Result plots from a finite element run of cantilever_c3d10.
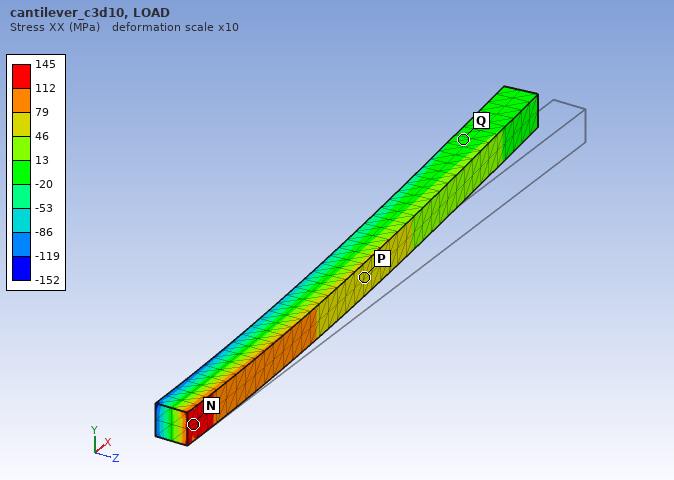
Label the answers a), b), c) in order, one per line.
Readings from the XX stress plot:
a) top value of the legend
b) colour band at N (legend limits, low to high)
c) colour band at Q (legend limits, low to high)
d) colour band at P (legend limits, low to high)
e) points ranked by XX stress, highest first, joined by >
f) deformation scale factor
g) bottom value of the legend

a) 145 MPa
b) 112 to 145 MPa
c) -20 to 13 MPa
d) 46 to 79 MPa
e) N > P > Q
f) 10
g) -152 MPa
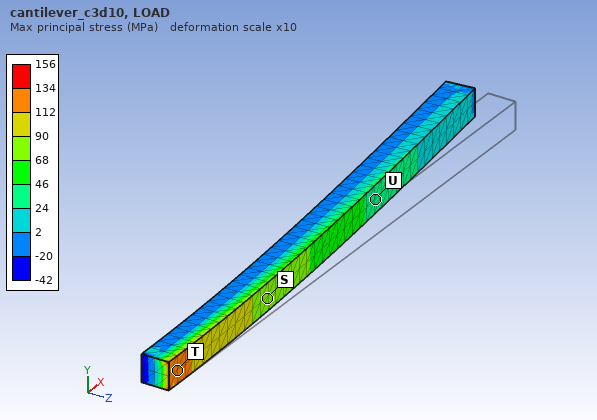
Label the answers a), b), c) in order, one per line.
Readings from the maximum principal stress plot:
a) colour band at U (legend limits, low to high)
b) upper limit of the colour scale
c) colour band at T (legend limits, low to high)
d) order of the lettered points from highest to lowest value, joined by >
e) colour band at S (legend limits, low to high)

a) 24 to 46 MPa
b) 156 MPa
c) 112 to 134 MPa
d) T > S > U
e) 68 to 90 MPa
